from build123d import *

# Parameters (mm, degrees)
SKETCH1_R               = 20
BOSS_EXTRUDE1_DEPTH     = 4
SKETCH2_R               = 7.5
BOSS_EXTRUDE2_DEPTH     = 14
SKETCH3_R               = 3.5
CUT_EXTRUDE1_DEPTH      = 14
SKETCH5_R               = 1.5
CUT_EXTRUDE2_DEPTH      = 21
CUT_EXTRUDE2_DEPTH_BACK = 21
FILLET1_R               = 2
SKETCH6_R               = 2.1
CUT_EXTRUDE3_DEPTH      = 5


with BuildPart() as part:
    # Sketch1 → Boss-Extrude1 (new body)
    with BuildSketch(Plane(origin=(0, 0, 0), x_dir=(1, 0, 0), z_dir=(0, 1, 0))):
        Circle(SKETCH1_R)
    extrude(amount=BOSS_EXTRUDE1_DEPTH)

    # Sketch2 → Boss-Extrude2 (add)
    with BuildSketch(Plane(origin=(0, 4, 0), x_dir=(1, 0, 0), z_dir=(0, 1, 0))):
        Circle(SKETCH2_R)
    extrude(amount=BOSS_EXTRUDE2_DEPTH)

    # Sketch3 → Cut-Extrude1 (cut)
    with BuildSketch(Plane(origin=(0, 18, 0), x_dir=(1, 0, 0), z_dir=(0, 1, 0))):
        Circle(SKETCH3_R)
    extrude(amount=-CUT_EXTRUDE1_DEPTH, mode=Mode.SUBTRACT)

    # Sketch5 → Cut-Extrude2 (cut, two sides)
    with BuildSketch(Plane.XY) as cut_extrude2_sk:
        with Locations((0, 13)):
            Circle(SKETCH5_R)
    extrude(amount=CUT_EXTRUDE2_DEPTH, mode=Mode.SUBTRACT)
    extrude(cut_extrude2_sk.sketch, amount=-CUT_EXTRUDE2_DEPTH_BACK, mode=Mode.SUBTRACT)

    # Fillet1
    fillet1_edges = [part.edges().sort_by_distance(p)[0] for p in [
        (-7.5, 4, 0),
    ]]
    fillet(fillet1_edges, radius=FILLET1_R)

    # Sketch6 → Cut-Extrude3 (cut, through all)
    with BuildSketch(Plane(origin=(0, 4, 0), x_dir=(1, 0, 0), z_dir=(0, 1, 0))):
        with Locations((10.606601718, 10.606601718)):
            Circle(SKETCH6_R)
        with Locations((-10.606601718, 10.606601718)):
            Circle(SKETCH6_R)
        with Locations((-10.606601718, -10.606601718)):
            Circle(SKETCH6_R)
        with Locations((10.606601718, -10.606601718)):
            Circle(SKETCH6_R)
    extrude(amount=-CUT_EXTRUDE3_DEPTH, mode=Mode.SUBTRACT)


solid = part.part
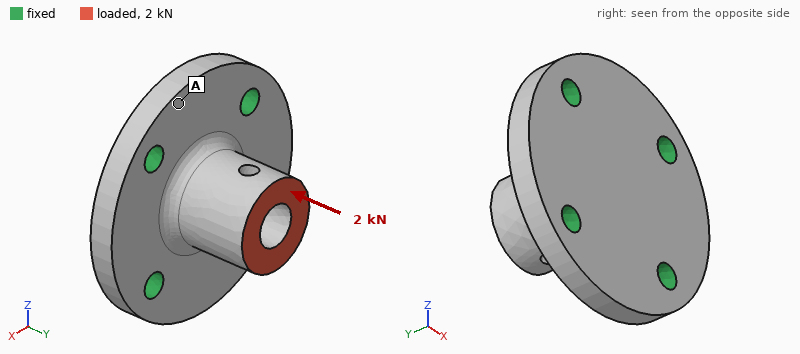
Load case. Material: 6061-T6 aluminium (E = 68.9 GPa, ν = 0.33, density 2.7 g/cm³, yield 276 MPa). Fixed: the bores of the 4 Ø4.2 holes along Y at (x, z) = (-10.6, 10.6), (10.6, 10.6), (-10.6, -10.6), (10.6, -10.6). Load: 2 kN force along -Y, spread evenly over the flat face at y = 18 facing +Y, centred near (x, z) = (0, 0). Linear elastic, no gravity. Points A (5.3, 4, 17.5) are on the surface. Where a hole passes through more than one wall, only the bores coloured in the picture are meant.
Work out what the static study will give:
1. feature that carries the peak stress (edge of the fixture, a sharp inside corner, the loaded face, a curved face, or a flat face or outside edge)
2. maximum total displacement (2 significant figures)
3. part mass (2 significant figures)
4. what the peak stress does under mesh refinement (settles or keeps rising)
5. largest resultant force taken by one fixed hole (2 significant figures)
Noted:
edge of the fixture
11 µm
18 g
keeps rising
520 N
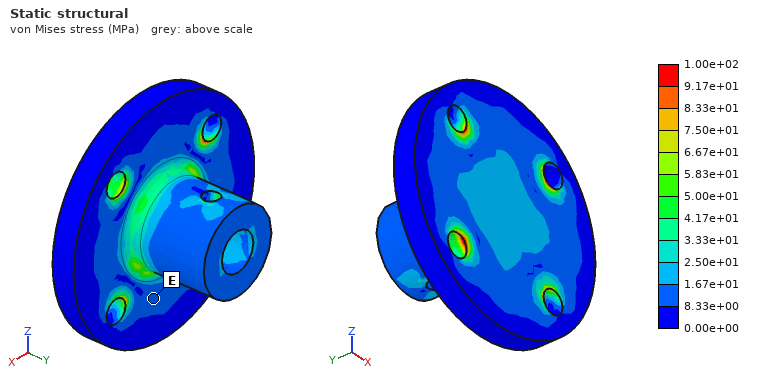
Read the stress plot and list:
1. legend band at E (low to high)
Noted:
8.33e+00 to 1.67e+01 MPa
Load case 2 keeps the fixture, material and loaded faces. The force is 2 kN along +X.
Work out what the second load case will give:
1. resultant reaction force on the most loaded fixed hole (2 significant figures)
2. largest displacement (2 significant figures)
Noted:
1.0 kN
58 µm
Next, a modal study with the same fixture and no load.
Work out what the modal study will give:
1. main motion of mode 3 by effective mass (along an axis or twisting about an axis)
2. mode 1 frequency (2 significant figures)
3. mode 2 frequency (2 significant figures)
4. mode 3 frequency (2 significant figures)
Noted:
along Y
22 kHz
22 kHz
27 kHz
